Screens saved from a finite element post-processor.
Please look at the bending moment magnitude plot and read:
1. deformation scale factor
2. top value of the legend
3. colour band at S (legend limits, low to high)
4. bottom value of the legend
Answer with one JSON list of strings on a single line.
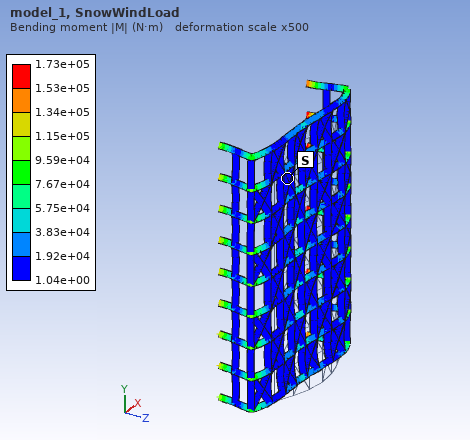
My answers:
["500", "1.73e+05 N·m", "1.04e+00 to 1.92e+04 N·m", "1.04e+00 N·m"]
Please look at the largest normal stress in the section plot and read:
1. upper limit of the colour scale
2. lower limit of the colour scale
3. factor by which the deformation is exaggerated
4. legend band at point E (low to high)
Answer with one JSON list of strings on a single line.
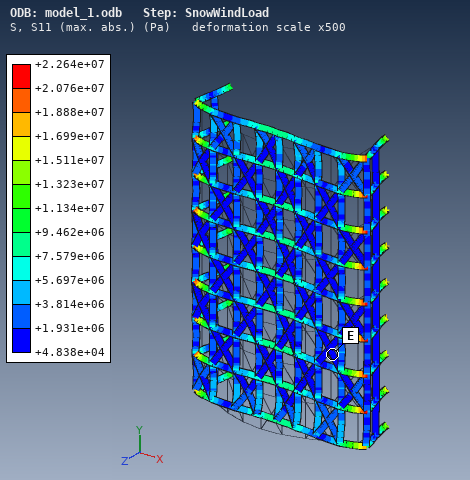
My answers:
["+2.264e+07 Pa", "+4.838e+04 Pa", "500", "+4.838e+04 to +1.931e+06 Pa"]
